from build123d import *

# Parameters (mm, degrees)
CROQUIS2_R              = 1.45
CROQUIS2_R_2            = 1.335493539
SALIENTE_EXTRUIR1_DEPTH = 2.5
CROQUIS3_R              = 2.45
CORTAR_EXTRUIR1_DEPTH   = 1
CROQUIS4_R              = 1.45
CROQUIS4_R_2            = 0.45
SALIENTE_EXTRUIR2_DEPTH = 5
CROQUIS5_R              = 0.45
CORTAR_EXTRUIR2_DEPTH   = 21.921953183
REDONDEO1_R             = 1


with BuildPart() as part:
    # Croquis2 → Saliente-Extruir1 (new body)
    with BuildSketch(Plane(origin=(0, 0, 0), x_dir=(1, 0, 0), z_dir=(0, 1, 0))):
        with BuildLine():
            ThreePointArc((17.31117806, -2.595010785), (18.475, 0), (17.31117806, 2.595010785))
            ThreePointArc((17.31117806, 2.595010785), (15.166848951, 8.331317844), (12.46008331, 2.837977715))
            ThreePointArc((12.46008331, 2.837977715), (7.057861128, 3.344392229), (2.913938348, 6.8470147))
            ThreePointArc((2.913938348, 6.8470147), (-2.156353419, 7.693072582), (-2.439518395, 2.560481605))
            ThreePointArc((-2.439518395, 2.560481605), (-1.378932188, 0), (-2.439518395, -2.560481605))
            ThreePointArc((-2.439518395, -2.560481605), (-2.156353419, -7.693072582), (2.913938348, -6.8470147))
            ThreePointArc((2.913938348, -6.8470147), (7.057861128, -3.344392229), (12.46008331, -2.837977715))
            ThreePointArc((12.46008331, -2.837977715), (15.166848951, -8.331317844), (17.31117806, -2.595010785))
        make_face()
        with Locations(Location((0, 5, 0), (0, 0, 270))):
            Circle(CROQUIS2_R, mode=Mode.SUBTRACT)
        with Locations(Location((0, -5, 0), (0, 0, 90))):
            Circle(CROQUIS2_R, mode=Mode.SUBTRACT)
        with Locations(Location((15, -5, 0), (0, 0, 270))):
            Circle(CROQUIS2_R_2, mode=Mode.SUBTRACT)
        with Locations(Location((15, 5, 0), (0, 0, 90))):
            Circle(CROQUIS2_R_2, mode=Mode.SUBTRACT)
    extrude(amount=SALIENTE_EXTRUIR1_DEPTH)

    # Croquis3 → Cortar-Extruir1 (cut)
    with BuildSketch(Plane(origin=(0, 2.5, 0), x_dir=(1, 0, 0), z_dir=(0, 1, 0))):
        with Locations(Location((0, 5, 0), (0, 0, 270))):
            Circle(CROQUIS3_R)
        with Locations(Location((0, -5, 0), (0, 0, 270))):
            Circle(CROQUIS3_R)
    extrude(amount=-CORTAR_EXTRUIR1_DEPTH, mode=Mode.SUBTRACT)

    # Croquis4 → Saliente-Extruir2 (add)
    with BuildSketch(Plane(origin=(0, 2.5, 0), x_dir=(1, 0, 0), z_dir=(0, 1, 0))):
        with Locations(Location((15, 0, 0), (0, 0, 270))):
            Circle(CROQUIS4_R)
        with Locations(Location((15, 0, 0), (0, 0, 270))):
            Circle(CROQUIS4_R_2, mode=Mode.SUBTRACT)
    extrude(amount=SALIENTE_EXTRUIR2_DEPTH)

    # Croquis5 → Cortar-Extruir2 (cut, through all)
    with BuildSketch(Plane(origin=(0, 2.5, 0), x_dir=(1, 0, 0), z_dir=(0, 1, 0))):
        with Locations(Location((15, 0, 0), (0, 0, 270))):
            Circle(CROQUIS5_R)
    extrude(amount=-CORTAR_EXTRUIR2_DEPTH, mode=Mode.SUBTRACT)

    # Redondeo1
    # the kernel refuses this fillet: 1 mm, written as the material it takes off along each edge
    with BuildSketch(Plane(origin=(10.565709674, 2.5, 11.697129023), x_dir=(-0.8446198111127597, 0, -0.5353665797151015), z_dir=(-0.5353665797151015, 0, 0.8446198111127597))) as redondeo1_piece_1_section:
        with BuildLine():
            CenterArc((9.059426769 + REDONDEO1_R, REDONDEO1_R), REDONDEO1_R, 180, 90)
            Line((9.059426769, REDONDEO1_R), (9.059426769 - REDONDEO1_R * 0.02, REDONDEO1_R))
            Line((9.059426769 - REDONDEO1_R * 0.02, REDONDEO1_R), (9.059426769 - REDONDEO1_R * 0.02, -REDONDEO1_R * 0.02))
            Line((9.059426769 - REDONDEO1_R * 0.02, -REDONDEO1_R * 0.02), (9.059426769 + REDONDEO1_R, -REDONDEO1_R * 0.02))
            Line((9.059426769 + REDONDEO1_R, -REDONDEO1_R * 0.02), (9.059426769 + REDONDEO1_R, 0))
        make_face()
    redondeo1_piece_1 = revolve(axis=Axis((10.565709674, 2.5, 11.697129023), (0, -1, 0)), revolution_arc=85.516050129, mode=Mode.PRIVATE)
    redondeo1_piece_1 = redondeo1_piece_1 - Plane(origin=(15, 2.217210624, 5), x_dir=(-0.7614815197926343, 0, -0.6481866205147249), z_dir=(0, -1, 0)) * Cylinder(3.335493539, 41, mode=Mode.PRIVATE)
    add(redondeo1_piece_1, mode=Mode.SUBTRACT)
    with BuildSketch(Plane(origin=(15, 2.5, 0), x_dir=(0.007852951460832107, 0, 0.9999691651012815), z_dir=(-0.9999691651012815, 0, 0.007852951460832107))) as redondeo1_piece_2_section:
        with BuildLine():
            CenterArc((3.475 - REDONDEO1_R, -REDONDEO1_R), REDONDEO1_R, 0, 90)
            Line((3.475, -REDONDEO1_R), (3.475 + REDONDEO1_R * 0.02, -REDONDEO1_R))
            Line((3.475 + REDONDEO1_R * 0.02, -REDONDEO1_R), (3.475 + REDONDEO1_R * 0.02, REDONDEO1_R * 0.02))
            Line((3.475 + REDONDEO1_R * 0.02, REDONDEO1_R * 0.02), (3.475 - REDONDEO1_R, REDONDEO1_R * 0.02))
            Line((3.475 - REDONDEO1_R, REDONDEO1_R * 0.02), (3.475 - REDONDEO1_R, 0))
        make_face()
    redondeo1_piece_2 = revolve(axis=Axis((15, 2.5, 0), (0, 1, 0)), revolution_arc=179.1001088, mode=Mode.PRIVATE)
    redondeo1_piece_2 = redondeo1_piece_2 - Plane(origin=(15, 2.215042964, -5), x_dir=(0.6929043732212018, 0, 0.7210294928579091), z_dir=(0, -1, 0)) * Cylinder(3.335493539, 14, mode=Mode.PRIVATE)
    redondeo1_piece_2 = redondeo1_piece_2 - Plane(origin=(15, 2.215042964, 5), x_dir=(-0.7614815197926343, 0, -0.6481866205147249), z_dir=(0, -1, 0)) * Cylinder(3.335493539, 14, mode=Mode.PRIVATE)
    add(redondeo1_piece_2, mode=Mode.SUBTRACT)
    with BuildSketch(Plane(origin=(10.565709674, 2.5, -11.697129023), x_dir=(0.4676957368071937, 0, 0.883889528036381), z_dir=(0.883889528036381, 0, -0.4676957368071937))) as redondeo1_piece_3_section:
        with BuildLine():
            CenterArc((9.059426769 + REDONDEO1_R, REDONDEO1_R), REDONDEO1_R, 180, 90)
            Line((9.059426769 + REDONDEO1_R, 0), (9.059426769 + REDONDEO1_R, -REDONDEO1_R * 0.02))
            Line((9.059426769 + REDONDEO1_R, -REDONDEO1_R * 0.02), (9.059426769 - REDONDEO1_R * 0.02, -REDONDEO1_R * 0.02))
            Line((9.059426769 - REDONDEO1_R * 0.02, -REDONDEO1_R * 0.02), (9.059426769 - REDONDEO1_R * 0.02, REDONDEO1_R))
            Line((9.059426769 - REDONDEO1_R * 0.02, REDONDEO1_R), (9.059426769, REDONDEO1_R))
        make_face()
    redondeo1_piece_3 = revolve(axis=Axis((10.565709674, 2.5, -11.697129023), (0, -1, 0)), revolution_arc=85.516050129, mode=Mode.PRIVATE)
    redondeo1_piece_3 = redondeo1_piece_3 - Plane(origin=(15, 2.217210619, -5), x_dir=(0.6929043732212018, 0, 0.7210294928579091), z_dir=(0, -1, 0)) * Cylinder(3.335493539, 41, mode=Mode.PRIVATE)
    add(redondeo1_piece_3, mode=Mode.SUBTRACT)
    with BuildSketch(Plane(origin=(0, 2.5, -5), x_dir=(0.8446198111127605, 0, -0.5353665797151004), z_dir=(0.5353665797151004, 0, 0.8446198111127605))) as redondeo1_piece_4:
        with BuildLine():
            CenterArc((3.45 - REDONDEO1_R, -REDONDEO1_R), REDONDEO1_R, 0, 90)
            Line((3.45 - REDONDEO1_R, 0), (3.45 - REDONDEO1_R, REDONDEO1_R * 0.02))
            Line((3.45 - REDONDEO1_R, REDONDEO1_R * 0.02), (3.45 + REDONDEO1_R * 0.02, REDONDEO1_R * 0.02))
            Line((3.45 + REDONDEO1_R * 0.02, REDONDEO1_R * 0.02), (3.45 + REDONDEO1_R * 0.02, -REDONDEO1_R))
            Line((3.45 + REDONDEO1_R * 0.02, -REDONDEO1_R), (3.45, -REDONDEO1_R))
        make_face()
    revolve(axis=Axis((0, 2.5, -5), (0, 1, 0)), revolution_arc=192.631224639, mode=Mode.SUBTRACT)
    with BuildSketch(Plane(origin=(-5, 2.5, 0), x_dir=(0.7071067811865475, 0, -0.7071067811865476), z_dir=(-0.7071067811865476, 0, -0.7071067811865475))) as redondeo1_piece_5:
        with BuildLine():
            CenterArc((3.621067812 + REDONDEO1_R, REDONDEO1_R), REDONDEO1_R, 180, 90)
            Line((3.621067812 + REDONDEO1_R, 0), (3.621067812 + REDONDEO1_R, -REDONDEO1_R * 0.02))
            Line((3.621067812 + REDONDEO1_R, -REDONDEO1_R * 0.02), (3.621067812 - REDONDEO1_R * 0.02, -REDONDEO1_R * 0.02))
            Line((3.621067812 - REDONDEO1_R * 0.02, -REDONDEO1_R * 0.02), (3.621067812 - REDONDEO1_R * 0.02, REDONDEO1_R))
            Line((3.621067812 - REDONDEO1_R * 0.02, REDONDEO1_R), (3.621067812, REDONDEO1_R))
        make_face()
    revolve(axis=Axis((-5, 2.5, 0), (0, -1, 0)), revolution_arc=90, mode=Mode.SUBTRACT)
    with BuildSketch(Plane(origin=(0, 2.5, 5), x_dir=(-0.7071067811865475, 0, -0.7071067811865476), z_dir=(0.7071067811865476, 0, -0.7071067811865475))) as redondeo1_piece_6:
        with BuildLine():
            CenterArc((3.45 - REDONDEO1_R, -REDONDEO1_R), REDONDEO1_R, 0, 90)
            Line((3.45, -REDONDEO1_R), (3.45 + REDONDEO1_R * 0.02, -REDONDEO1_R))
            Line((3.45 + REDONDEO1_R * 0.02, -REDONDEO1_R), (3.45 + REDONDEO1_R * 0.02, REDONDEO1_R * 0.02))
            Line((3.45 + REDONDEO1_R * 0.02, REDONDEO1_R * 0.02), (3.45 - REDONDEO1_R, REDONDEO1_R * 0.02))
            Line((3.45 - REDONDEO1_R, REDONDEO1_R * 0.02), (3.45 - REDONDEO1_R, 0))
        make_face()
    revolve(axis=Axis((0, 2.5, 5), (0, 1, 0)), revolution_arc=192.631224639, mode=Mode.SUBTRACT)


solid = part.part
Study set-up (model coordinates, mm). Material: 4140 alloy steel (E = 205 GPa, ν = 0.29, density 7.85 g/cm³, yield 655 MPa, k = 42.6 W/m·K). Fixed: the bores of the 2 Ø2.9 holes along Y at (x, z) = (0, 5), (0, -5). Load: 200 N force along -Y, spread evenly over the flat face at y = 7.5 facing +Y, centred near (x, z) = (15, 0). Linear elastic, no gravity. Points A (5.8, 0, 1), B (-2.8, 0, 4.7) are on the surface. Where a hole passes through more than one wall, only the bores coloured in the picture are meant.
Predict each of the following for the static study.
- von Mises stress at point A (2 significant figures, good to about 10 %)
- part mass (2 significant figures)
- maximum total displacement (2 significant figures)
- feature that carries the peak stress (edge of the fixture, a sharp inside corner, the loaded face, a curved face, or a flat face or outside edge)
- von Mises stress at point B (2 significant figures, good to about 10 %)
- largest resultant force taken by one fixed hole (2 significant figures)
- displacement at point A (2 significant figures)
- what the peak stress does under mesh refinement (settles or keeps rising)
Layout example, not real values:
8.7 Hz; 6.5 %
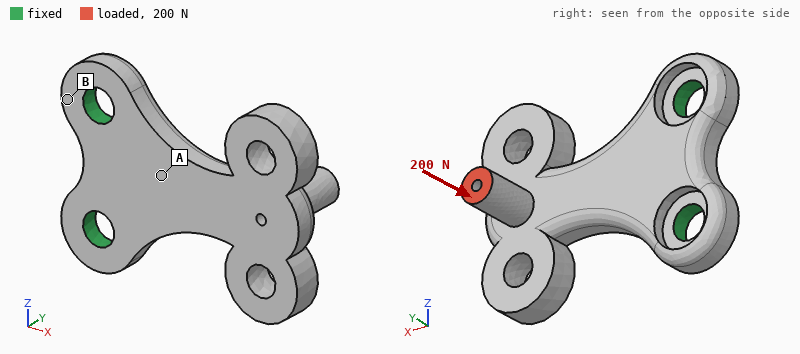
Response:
260 MPa; 4.4 g; 0.17 mm; edge of the fixture; 57 MPa; 110 N; 0.026 mm; keeps rising
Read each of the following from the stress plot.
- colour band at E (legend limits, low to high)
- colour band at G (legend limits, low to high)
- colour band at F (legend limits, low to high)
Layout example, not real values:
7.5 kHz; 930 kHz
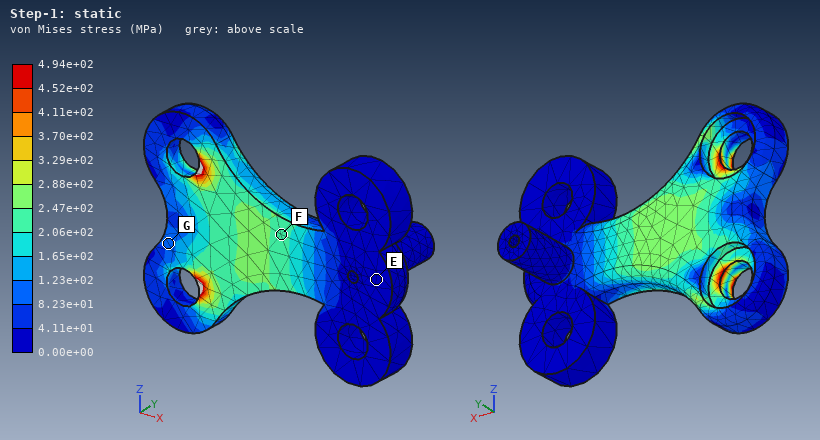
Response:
0.00e+00 to 4.11e+01 MPa; 8.23e+01 to 1.23e+02 MPa; 2.06e+02 to 2.47e+02 MPa
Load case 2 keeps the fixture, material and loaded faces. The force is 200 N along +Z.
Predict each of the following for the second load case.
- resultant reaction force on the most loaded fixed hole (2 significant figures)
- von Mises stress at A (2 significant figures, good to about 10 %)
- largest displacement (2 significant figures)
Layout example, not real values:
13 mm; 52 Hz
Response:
340 N; 160 MPa; 77 µm
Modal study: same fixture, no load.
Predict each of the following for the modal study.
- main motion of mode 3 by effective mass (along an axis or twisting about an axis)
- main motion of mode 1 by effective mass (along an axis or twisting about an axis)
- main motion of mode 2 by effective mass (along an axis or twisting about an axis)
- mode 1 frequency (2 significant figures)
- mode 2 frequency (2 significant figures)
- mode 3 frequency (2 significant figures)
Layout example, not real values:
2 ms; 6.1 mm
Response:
along Z; along Y; twisting about X; 4400 Hz; 11 kHz; 13 kHz
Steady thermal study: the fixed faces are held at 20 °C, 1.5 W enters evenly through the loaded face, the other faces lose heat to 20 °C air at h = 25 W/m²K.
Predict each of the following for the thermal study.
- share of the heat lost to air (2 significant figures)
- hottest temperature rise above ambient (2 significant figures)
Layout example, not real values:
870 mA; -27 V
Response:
19 %; 57 K
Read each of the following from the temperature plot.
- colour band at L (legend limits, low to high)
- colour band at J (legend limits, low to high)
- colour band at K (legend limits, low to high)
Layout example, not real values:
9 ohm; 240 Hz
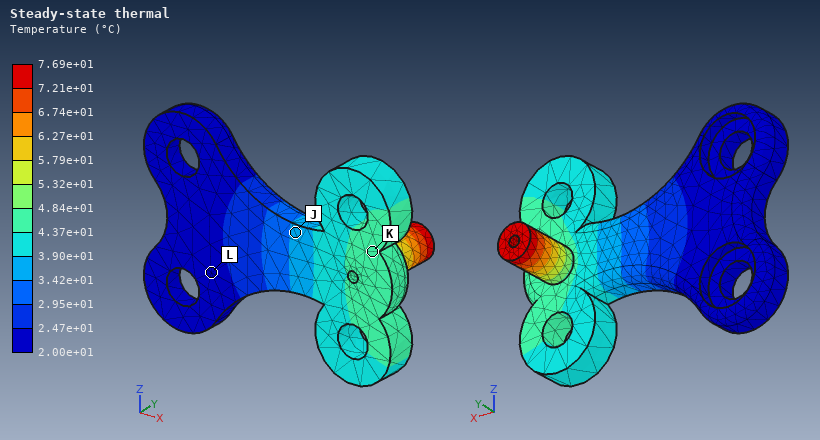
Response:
2.00e+01 to 2.47e+01 °C; 3.42e+01 to 3.90e+01 °C; 4.37e+01 to 4.84e+01 °C
